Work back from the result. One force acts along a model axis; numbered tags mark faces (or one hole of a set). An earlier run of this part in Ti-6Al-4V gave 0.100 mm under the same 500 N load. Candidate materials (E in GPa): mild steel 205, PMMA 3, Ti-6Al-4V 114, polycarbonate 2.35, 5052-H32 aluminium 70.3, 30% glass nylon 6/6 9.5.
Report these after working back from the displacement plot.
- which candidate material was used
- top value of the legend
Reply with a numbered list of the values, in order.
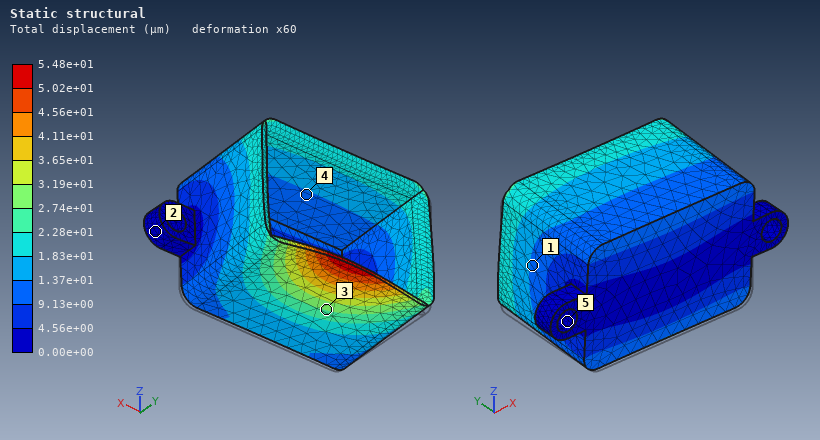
1. mild steel
2. 5.48e+01 µm
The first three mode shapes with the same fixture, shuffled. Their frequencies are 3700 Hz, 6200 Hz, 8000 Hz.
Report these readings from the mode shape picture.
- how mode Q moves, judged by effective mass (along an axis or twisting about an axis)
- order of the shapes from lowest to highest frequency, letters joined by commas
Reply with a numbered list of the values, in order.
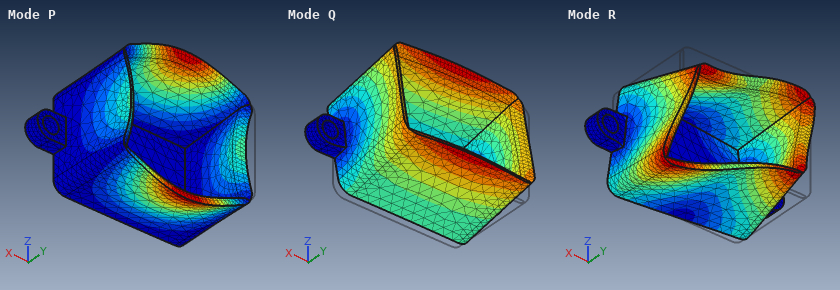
1. along Z
2. Q, R, P
